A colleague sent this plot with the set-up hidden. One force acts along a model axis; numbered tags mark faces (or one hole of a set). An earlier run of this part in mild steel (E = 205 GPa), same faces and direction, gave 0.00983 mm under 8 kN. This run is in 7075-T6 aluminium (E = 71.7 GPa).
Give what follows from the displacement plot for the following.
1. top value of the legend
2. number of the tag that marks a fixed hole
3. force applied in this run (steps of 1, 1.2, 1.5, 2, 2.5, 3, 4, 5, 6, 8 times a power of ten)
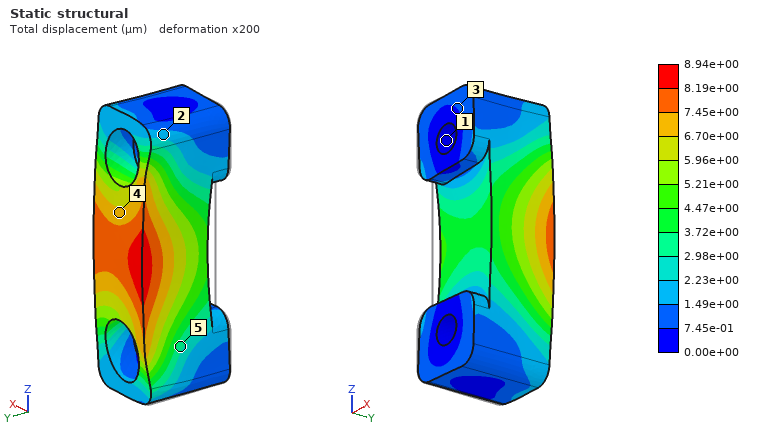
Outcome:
8.94e+00 µm
1
2.5 kN
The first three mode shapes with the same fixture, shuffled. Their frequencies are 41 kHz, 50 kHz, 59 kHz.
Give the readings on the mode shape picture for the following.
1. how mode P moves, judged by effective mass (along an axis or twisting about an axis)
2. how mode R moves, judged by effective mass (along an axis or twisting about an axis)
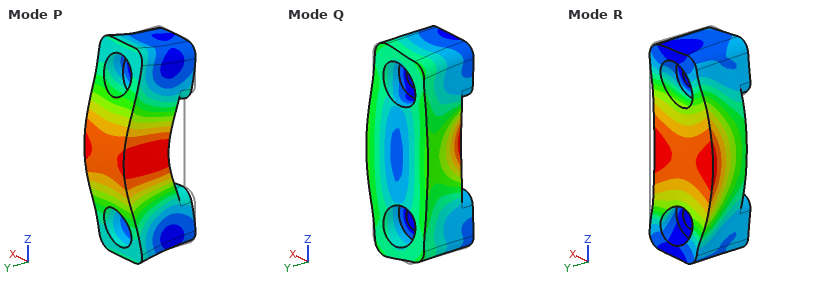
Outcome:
along Y
along X
